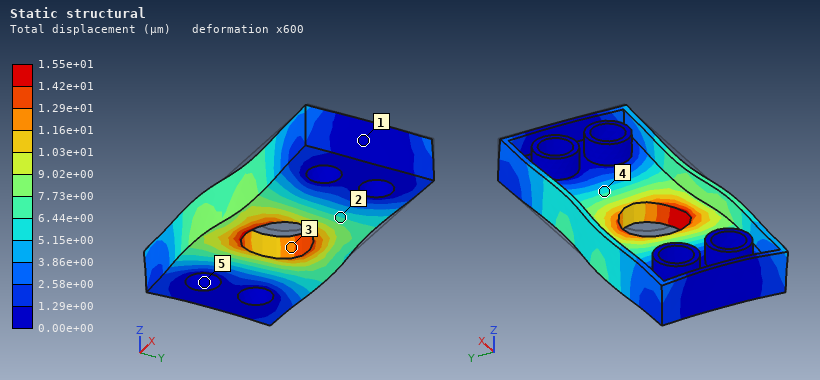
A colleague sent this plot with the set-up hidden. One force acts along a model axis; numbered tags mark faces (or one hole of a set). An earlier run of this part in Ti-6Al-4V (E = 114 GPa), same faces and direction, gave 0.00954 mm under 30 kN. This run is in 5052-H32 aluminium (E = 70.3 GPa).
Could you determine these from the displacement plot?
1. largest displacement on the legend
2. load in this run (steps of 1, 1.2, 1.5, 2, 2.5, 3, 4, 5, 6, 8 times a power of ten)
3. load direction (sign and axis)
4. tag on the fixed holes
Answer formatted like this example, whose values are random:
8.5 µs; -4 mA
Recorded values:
1.55e+01 µm; 30 kN; -X; 5
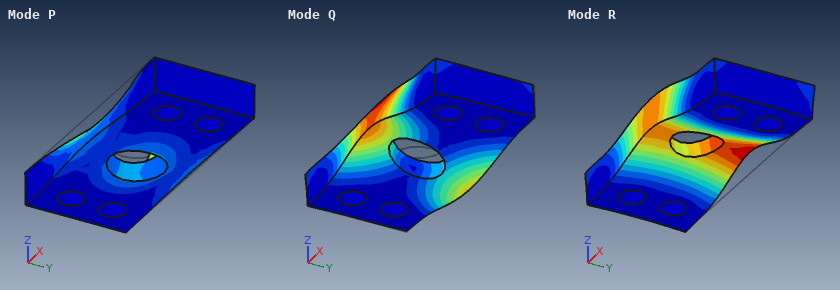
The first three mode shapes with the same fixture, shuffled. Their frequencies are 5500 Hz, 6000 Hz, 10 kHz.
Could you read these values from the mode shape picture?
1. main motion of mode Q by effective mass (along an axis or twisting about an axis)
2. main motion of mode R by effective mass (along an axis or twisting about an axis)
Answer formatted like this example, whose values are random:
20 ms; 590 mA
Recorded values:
twisting about X; along Z
